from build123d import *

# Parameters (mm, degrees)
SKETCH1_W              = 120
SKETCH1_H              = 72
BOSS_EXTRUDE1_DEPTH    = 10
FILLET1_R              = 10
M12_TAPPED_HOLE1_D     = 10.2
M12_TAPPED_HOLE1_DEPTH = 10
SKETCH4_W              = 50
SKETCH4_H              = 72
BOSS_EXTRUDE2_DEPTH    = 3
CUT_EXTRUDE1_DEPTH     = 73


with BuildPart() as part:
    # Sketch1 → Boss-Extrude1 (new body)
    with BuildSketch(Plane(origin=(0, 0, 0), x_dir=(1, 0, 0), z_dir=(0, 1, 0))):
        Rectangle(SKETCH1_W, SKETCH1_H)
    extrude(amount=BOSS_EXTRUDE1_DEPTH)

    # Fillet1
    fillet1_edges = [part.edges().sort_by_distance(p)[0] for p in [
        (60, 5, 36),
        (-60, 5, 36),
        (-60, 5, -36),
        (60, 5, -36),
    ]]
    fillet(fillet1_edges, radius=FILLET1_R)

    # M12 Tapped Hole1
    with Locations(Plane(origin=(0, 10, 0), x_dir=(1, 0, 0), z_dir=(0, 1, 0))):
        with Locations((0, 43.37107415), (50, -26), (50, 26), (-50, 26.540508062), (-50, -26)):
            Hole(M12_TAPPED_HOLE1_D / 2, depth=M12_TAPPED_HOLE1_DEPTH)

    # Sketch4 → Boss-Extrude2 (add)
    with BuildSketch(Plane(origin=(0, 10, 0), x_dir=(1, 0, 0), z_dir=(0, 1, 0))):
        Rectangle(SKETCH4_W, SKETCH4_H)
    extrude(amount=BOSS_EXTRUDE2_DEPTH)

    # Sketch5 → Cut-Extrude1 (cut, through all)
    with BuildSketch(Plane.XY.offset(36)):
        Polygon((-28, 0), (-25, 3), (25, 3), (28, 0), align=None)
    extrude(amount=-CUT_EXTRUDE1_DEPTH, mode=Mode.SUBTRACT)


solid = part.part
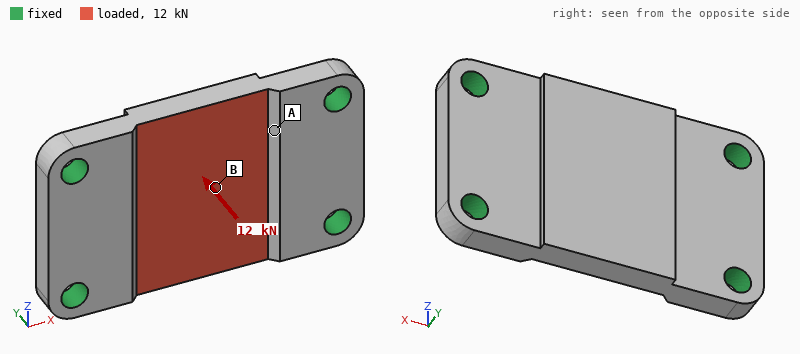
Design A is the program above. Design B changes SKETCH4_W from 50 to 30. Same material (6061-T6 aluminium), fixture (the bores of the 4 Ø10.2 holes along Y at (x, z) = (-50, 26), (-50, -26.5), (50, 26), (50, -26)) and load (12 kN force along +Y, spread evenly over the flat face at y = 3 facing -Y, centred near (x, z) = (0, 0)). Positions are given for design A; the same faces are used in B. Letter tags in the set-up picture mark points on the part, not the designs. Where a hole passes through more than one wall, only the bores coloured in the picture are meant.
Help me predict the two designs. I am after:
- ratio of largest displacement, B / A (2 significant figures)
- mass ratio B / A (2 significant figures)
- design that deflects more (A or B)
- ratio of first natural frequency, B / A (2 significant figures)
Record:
1.1
0.95
B
0.97
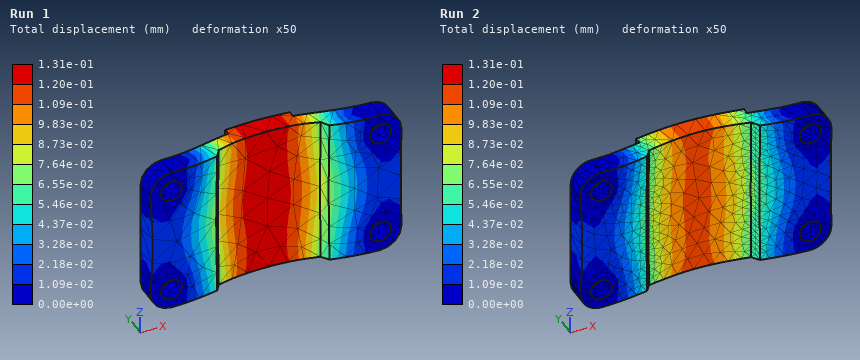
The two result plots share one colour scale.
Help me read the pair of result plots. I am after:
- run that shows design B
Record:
Run 1
